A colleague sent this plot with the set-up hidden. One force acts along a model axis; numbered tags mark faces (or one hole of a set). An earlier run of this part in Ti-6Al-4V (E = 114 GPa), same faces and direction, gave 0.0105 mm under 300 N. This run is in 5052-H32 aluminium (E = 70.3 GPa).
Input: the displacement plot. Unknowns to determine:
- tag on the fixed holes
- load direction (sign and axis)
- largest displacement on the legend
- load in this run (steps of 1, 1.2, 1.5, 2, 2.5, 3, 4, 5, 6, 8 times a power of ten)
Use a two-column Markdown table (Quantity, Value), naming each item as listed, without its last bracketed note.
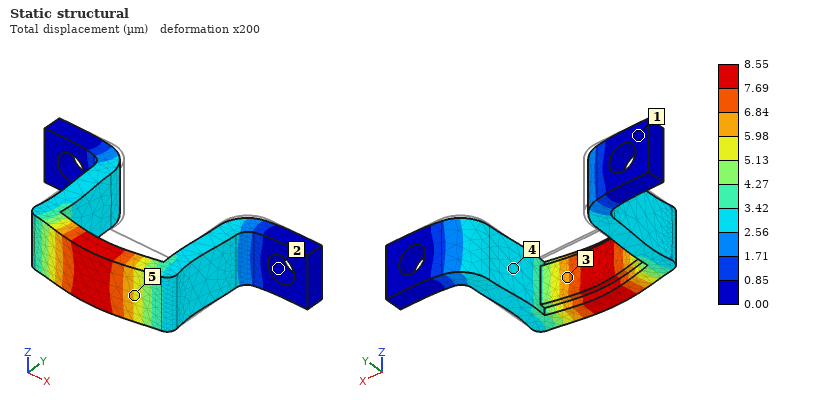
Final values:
| Quantity | Value |
|---|---|
| tag on the fixed holes | 2 |
| load direction | -Y |
| largest displacement on the legend | 8.55 µm |
| load in this run | 150 N |
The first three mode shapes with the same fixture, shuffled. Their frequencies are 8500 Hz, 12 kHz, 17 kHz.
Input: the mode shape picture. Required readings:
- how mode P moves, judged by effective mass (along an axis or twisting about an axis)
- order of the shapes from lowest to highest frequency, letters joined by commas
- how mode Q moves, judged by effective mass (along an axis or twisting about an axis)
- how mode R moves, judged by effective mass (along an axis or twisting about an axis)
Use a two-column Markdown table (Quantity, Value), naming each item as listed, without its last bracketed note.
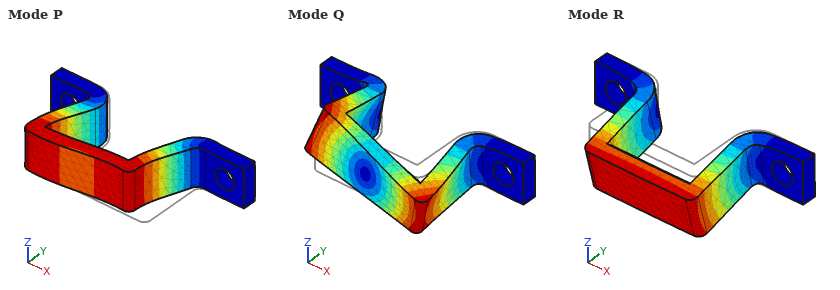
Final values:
| Quantity | Value |
|---|---|
| how mode P moves, judged by effective mass | along X |
| order of the shapes from lowest to highest frequency, letters joined by commas | R, P, Q |
| how mode Q moves, judged by effective mass | twisting about Y |
| how mode R moves, judged by effective mass | along Z |
